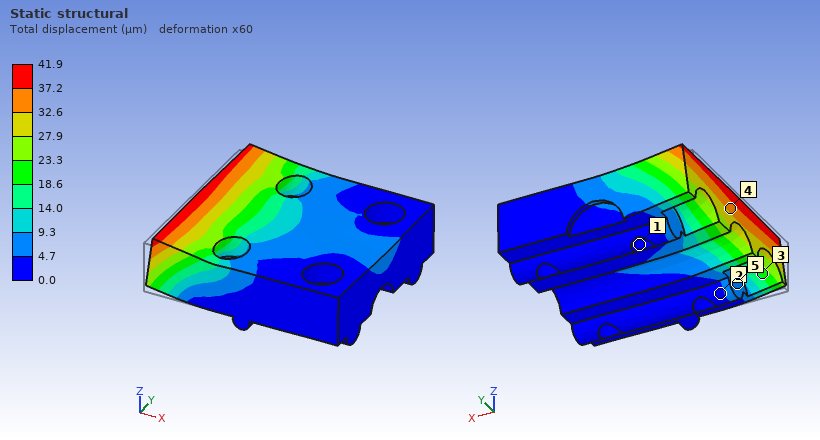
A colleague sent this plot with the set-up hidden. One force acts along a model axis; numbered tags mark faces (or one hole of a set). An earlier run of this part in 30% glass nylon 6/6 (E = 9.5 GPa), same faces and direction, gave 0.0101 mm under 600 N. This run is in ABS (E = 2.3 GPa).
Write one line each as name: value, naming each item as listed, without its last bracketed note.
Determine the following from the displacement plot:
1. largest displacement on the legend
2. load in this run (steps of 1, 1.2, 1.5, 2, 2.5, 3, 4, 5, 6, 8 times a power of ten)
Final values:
largest displacement on the legend: 41.9 µm
load in this run: 600 N
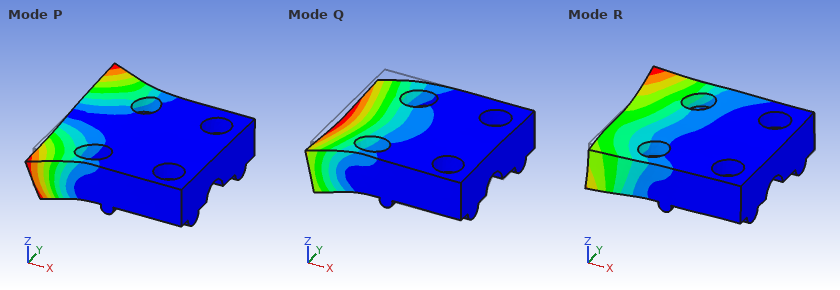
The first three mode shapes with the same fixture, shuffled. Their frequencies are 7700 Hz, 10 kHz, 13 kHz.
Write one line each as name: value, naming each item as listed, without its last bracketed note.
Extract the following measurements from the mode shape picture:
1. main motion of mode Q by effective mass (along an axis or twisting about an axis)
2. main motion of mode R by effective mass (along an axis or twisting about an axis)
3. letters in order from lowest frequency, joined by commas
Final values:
main motion of mode Q by effective mass: along Z
main motion of mode R by effective mass: along Y
letters in order from lowest frequency, joined by commas: Q, P, R
